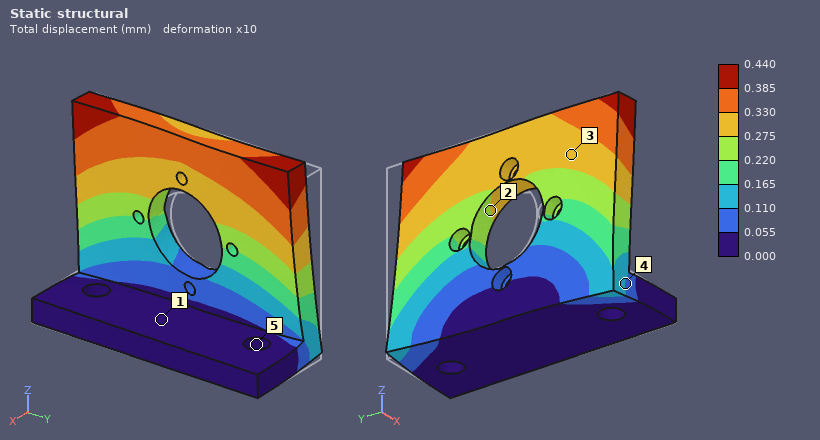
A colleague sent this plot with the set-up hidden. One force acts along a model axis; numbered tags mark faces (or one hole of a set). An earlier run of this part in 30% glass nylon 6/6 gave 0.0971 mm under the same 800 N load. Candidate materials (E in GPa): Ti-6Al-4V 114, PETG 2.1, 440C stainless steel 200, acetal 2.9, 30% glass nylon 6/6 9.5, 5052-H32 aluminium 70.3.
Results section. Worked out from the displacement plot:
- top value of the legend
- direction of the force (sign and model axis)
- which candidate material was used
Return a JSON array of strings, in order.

["0.440 mm", "-Y", "PETG"]
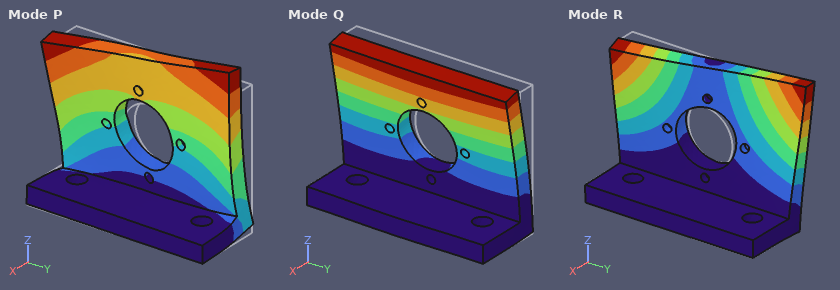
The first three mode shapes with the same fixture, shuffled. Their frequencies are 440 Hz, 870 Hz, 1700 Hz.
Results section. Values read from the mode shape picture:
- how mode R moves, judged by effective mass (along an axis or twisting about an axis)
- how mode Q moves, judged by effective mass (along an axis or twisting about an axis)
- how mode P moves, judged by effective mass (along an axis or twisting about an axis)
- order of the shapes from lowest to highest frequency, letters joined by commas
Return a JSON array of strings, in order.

["twisting about Z", "along X", "along Y", "Q, R, P"]
